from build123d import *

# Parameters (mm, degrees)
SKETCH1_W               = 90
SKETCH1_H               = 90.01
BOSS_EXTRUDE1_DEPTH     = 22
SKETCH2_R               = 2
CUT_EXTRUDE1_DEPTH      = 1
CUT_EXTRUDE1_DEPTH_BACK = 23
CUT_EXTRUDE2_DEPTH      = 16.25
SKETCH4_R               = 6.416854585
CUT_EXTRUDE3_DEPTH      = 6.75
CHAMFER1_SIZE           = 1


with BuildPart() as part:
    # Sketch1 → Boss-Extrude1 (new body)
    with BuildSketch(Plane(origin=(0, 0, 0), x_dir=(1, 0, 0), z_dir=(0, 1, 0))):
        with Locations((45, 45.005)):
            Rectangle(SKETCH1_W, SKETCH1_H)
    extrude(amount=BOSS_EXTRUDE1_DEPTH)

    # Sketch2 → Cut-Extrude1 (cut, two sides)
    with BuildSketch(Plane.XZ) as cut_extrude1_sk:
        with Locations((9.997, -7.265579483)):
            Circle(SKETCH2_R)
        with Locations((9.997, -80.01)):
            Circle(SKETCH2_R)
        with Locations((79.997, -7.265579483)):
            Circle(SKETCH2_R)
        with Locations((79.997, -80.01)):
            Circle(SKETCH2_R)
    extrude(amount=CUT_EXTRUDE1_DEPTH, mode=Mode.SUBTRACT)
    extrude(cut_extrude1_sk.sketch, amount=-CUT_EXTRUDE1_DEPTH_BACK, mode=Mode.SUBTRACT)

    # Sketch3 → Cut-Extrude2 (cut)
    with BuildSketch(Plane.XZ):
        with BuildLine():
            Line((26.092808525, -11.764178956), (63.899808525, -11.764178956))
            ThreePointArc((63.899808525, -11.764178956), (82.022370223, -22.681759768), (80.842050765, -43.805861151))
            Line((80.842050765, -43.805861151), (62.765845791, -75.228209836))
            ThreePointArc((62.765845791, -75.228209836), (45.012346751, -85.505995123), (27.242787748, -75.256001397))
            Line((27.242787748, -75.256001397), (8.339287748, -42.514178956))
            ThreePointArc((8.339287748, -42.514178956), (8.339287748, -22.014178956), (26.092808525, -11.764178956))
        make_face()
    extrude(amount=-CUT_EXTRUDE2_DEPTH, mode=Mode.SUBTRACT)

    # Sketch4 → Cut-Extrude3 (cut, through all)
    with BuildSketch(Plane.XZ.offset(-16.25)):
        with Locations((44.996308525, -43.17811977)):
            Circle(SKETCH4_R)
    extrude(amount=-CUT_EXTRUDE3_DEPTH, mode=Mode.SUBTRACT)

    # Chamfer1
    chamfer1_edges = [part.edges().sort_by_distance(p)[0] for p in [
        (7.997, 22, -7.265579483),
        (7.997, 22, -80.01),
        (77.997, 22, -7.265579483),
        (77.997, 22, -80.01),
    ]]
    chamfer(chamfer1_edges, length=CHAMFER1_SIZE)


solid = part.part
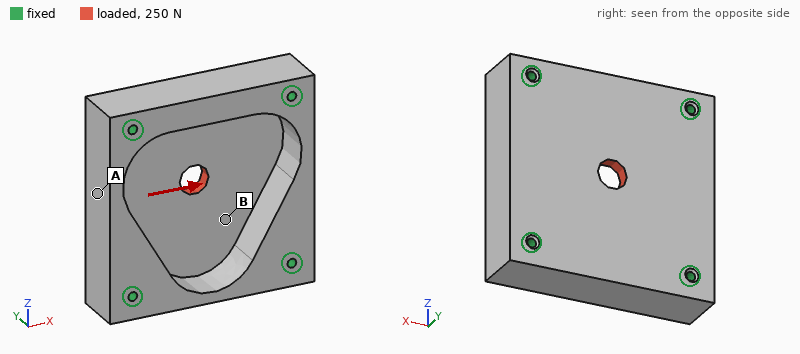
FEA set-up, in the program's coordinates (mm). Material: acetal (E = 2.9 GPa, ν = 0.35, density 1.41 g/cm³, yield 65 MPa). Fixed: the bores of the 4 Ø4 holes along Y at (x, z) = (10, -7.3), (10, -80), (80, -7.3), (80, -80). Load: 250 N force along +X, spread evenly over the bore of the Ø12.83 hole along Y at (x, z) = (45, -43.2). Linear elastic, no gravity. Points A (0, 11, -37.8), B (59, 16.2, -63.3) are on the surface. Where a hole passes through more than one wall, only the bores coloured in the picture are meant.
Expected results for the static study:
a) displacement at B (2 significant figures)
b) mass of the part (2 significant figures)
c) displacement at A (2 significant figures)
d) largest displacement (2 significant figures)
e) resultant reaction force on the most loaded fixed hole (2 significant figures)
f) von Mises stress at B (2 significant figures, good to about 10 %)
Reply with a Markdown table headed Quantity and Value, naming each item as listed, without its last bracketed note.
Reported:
| Quantity | Value |
|---|---|
| displacement at B | 5.0 µm |
| mass of the part | 150 g |
| displacement at A | 4.2 µm |
| largest displacement | 11 µm |
| resultant reaction force on the most loaded fixed hole | 68 N |
| von Mises stress at B | 0.55 MPa |
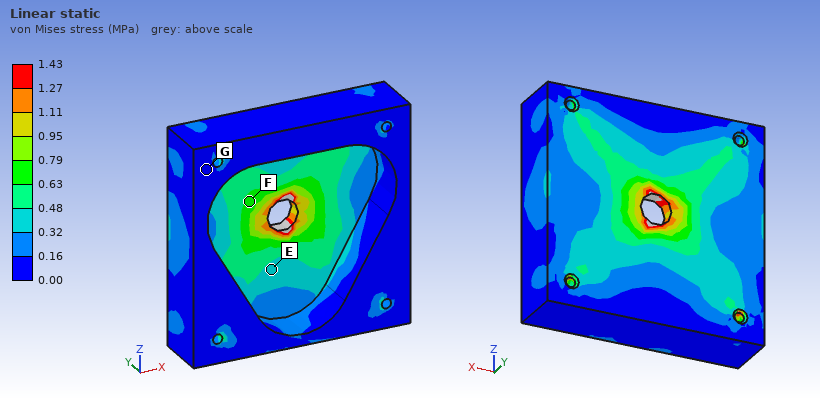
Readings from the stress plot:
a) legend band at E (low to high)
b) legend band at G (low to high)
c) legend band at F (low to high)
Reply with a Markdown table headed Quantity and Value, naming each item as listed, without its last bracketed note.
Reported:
| Quantity | Value |
|---|---|
| legend band at E | 0.32 to 0.48 MPa |
| legend band at G | 0.00 to 0.16 MPa |
| legend band at F | 0.63 to 0.79 MPa |
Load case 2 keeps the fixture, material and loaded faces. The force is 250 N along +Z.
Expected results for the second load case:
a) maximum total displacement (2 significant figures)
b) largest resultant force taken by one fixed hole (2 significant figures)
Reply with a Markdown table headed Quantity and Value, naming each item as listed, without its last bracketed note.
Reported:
| Quantity | Value |
|---|---|
| maximum total displacement | 11 µm |
| largest resultant force taken by one fixed hole | 73 N |
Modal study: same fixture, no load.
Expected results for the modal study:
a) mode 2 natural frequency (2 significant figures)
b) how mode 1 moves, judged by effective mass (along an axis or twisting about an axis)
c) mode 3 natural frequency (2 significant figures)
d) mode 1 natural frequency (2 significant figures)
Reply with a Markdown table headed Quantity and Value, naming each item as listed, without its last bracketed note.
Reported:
| Quantity | Value |
|---|---|
| mode 2 natural frequency | 3600 Hz |
| how mode 1 moves, judged by effective mass | along Y |
| mode 3 natural frequency | 3700 Hz |
| mode 1 natural frequency | 2300 Hz |
